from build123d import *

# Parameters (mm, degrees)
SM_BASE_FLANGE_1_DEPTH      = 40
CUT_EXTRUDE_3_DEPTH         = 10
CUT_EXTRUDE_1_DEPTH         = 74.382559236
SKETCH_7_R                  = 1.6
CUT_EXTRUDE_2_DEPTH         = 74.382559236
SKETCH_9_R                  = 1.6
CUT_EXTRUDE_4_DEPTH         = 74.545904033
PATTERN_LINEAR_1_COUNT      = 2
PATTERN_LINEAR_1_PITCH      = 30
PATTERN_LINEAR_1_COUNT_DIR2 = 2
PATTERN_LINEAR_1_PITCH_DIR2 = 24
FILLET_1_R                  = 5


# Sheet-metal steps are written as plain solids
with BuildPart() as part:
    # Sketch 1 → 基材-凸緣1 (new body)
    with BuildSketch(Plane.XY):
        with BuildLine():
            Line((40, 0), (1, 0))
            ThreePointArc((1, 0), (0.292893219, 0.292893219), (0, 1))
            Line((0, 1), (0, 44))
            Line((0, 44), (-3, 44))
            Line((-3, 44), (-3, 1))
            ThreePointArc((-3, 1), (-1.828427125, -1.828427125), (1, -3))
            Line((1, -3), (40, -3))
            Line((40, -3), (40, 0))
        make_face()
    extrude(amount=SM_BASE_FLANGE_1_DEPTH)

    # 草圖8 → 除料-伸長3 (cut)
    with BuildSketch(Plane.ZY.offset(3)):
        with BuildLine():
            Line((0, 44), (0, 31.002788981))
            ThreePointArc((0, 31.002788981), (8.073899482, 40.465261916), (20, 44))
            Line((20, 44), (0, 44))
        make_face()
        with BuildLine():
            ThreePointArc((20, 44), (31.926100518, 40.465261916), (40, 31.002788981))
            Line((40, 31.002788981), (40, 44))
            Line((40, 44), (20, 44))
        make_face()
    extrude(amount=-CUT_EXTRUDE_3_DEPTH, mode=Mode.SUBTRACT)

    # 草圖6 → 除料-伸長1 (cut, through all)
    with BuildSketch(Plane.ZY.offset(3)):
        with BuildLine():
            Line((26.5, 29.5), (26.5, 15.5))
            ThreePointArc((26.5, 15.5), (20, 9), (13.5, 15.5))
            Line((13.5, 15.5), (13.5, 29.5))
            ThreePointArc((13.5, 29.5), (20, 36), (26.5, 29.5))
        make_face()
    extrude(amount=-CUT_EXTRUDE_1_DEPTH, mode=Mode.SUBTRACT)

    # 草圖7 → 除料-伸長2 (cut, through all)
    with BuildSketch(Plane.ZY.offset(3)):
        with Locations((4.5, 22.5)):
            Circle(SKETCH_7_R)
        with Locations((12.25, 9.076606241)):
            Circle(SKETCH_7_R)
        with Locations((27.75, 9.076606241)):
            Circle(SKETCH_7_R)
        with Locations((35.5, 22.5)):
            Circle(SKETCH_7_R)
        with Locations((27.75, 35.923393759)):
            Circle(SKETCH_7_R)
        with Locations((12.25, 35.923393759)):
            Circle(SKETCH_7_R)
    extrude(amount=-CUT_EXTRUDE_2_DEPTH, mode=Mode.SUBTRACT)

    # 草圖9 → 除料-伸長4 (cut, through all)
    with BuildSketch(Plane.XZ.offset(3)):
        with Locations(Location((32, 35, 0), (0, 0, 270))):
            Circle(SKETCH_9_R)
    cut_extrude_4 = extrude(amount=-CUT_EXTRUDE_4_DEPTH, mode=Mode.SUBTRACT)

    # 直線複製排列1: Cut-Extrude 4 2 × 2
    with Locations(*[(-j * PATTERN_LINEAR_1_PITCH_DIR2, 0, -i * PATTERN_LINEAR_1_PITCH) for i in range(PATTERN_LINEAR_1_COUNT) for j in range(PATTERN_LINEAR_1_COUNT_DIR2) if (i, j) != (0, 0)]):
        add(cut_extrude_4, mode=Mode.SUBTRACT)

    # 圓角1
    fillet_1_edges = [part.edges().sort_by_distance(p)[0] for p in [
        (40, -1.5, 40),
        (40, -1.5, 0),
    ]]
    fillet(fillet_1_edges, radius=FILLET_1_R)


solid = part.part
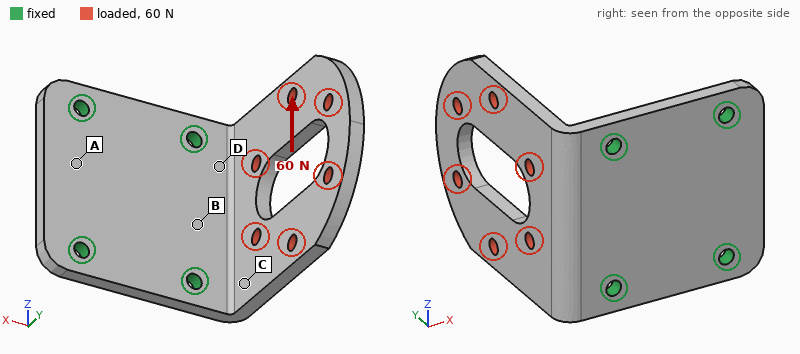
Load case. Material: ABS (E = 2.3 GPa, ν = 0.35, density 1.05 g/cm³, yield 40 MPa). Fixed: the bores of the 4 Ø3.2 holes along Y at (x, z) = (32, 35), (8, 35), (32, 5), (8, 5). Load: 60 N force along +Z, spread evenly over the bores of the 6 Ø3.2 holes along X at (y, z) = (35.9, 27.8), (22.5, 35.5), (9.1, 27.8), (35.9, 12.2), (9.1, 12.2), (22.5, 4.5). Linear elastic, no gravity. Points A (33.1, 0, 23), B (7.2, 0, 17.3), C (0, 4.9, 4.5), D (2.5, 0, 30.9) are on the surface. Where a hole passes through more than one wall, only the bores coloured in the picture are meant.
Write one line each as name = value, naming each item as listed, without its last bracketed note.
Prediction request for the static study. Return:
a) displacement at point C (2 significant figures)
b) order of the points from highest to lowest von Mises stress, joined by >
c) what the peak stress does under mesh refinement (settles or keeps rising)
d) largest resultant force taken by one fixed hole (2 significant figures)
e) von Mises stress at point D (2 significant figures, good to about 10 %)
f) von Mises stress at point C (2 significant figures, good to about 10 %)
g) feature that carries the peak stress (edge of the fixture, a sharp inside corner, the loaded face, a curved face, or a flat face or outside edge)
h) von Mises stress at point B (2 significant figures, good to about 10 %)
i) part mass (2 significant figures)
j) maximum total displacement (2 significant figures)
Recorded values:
displacement at point C = 0.14 mm
order of the points from highest to lowest von Mises stress, joined by > = D > C > B > A
what the peak stress does under mesh refinement = keeps rising
largest resultant force taken by one fixed hole = 59 N
von Mises stress at point D = 6.2 MPa
von Mises stress at point C = 4.5 MPa
feature that carries the peak stress = edge of the fixture
von Mises stress at point B = 2.4 MPa
part mass = 9.1 g
maximum total displacement = 0.44 mm
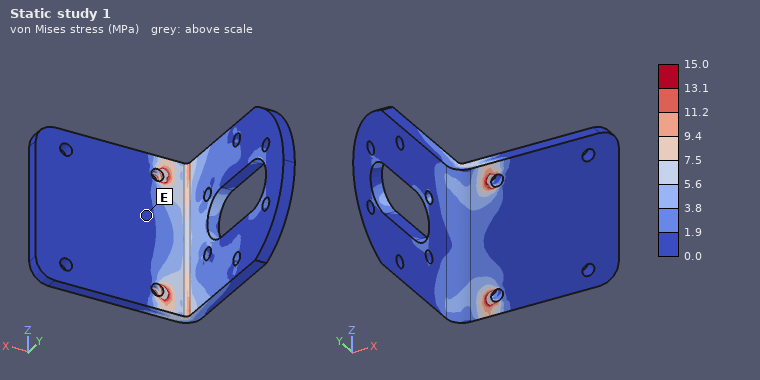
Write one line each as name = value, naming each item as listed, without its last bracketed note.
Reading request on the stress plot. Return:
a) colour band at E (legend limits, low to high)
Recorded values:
colour band at E = 0.0 to 1.9 MPa
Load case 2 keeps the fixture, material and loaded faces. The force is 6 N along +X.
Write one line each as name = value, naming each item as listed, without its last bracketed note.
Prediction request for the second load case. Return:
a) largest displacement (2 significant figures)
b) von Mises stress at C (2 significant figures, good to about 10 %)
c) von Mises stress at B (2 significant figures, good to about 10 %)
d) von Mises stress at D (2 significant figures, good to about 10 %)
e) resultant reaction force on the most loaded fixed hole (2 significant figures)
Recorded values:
largest displacement = 0.70 mm
von Mises stress at C = 1.9 MPa
von Mises stress at B = 1.3 MPa
von Mises stress at D = 2.2 MPa
resultant reaction force on the most loaded fixed hole = 2.2 N
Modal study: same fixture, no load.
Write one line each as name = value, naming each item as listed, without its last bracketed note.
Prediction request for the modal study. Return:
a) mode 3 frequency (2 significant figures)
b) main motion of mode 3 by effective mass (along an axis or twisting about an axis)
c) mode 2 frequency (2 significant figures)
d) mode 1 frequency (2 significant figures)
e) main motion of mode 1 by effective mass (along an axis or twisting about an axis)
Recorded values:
mode 3 frequency = 1300 Hz
main motion of mode 3 by effective mass = along Z
mode 2 frequency = 840 Hz
mode 1 frequency = 320 Hz
main motion of mode 1 by effective mass = along X
